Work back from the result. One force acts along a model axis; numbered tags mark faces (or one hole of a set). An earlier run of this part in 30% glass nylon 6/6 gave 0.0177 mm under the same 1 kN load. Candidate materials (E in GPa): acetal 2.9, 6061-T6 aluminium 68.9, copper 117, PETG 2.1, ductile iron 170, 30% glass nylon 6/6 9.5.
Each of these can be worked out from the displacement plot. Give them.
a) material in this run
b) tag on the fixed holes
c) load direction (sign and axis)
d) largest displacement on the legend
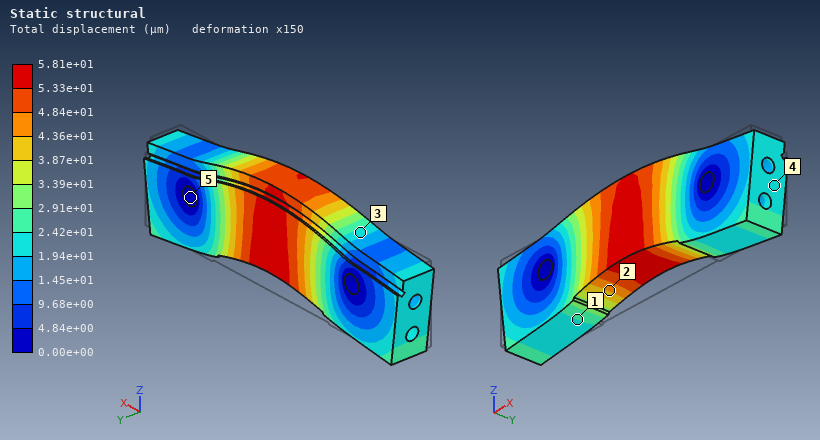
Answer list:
acetal
5
+Z
5.81e+01 µm
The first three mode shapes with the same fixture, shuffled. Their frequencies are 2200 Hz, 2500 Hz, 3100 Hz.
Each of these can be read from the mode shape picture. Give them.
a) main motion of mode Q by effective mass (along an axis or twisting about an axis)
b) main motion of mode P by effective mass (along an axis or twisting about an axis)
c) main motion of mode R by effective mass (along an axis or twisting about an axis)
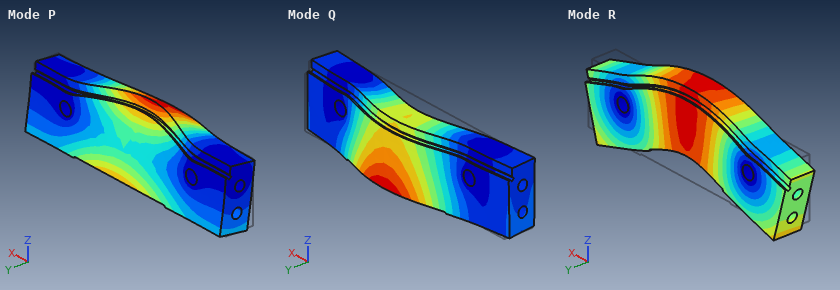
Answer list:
along Y
twisting about X
along Z
